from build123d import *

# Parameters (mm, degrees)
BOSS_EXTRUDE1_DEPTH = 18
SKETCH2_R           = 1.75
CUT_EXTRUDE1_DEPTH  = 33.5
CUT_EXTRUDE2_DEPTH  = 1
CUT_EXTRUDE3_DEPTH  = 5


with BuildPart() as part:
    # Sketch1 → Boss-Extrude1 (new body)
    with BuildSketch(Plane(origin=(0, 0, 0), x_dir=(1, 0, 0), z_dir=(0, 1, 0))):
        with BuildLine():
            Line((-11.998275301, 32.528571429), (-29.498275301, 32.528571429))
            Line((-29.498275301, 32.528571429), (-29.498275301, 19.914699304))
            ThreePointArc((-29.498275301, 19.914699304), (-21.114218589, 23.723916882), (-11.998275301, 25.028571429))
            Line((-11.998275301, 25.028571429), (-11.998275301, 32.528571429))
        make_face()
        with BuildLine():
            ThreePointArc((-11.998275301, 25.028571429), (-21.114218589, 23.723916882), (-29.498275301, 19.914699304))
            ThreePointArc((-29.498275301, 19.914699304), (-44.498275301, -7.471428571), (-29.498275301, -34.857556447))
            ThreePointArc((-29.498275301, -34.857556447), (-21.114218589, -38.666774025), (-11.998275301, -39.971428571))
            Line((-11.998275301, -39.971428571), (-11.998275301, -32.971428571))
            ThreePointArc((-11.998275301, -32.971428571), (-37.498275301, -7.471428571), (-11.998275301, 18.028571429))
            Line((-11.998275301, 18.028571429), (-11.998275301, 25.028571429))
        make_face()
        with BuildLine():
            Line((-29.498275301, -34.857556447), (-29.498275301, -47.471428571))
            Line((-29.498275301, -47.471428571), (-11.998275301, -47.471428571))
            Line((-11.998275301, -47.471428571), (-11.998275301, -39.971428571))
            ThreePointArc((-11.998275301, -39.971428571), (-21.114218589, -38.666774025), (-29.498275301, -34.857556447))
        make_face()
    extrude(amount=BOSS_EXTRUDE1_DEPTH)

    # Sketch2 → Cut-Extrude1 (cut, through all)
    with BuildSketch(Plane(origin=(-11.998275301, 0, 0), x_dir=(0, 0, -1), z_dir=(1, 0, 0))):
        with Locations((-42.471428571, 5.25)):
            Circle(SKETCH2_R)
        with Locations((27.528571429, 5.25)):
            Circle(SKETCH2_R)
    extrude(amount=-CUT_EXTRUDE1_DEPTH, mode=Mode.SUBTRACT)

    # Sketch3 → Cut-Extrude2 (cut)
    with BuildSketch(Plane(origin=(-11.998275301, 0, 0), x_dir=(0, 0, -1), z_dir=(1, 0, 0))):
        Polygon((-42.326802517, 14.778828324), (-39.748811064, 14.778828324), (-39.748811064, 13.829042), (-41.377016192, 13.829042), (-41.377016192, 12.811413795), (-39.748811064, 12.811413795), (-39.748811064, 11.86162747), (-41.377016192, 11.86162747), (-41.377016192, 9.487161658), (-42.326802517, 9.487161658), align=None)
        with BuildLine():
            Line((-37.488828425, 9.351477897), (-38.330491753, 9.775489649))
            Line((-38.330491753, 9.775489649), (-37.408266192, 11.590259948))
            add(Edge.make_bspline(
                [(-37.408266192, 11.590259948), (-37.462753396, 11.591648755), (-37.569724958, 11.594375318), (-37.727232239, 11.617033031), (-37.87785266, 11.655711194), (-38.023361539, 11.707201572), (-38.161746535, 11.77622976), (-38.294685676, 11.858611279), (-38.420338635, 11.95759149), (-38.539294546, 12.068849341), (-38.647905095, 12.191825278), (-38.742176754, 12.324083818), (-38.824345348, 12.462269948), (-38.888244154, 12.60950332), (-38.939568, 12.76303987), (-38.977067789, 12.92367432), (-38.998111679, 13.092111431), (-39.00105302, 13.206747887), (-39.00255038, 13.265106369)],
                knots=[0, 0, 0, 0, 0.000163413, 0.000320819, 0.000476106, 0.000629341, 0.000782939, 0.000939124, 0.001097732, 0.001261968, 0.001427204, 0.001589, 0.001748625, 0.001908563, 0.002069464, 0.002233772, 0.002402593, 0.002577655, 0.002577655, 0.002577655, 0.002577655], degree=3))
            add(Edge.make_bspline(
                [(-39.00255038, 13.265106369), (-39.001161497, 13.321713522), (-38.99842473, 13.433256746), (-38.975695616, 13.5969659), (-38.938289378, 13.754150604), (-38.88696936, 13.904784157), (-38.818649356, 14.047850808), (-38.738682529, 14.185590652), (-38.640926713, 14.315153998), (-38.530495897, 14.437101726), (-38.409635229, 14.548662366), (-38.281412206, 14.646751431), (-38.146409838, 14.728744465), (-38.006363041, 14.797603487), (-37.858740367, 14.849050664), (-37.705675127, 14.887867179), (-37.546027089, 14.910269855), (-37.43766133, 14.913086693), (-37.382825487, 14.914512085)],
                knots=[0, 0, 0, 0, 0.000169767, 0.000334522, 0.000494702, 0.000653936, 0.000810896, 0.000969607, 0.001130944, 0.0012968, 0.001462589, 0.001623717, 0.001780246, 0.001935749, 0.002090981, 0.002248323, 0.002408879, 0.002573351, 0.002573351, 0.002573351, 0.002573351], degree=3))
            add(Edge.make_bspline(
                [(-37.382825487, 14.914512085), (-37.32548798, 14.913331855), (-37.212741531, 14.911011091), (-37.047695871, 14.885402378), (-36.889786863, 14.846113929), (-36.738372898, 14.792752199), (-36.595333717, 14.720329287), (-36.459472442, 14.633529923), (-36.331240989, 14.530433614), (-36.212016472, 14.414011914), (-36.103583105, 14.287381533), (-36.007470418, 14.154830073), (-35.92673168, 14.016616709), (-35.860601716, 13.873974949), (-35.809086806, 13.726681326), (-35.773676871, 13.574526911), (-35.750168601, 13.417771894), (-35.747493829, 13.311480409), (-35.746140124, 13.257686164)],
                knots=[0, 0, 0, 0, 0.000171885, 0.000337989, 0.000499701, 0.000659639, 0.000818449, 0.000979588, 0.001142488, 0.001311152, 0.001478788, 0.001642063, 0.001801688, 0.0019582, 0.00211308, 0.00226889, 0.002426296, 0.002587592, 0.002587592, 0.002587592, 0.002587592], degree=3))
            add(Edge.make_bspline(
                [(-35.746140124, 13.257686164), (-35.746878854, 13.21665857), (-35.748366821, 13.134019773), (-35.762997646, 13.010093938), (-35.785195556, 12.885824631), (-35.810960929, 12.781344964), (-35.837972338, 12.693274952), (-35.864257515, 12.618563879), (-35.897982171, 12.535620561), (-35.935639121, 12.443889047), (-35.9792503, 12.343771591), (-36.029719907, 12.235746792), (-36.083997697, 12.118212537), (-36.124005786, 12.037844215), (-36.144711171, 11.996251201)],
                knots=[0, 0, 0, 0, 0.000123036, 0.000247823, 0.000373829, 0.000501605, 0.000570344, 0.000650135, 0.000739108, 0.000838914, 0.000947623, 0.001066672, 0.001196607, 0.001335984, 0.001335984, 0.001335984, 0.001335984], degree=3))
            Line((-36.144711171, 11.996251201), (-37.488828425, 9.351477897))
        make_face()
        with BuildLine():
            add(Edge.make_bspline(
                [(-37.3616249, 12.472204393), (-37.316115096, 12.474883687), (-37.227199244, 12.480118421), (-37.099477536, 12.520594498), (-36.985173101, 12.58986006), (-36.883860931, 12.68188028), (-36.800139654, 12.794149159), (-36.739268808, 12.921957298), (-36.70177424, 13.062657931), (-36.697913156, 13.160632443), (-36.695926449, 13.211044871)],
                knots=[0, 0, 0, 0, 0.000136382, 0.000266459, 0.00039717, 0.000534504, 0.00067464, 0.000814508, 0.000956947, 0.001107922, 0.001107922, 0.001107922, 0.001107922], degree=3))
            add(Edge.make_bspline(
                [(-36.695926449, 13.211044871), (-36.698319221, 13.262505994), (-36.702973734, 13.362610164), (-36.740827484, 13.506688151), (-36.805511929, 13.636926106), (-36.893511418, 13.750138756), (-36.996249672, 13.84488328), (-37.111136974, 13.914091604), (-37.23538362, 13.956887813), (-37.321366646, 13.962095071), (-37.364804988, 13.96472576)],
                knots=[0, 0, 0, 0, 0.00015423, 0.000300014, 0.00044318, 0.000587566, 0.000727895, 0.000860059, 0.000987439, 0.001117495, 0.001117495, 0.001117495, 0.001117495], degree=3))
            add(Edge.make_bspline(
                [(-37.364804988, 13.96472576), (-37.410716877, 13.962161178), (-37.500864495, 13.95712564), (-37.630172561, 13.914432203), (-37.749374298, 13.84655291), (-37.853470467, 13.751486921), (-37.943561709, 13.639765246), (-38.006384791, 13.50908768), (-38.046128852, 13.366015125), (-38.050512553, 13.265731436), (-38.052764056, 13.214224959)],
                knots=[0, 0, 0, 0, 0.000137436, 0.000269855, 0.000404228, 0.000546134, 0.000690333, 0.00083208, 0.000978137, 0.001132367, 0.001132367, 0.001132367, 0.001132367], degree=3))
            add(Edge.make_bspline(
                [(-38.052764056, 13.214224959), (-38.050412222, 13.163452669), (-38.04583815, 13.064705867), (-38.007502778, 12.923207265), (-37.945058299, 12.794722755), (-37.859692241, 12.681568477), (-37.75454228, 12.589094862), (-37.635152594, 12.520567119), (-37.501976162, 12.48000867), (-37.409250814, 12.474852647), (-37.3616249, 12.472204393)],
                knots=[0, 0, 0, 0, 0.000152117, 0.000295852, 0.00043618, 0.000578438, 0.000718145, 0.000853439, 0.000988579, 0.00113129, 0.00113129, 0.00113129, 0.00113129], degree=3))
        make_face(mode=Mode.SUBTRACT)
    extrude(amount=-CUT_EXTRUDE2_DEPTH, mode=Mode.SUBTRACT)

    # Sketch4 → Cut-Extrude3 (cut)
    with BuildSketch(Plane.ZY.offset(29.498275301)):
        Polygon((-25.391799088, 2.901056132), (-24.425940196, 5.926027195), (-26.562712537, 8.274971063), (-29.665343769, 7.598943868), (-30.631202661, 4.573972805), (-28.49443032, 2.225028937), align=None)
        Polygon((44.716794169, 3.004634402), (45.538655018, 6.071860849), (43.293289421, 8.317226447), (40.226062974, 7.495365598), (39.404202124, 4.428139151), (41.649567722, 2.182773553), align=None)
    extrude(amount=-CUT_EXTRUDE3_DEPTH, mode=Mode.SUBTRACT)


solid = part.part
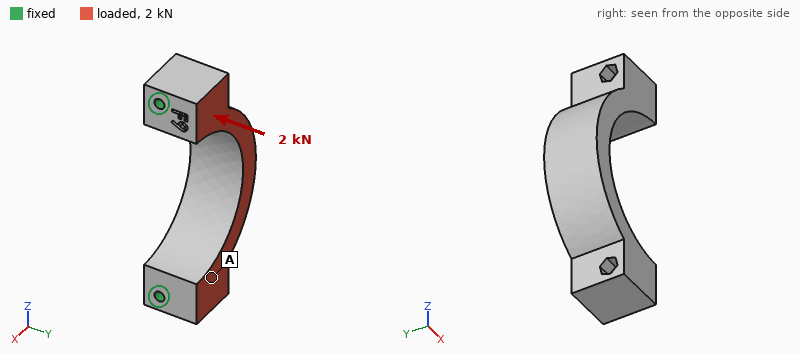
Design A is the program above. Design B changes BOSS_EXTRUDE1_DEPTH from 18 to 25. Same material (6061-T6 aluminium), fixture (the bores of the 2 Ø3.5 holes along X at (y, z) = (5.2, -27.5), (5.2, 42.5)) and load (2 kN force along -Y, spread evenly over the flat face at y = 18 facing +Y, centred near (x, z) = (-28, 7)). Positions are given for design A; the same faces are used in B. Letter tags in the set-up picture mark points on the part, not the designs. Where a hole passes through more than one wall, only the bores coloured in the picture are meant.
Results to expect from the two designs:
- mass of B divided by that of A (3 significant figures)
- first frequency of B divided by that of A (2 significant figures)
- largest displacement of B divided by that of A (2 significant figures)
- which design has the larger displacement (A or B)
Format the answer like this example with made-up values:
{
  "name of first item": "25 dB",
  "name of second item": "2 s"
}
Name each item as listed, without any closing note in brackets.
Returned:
{
  "mass of B divided by that of A": "1.40",
  "first frequency of B divided by that of A": "0.88",
  "largest displacement of B divided by that of A": "0.87",
  "which design has the larger displacement": "A"
}
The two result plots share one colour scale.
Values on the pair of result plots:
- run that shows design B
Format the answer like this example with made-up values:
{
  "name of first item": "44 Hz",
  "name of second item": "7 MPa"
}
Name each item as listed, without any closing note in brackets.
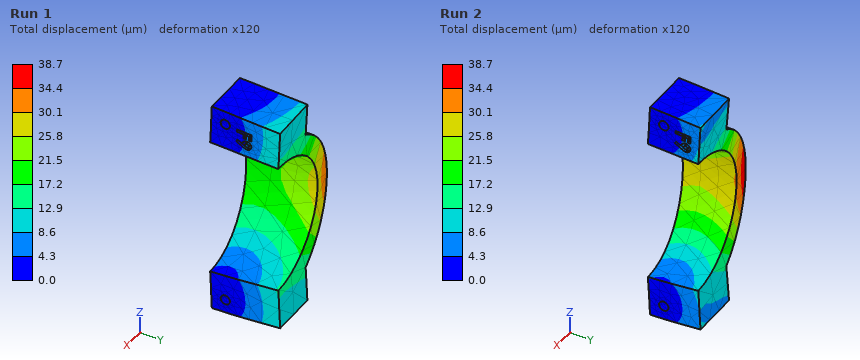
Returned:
{
  "run that shows design B": "Run 1"
}
